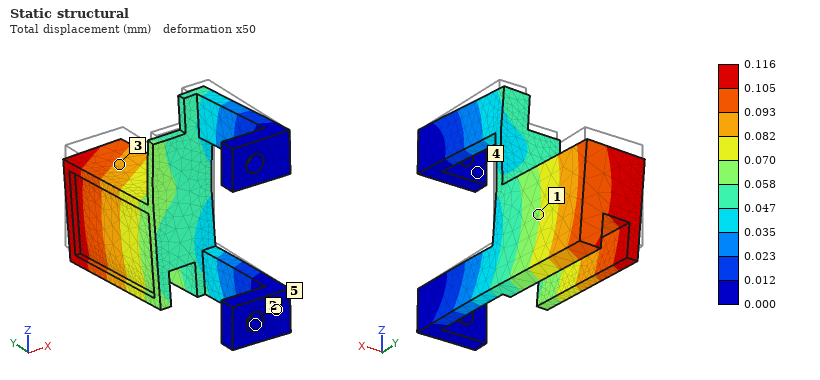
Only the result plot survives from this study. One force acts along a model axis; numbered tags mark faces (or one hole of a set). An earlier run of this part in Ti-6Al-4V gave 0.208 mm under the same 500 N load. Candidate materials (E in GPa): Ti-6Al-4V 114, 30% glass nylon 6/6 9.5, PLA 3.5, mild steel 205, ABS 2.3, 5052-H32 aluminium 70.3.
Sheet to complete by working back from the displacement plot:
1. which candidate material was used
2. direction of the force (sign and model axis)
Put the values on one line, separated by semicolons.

mild steel; -Z
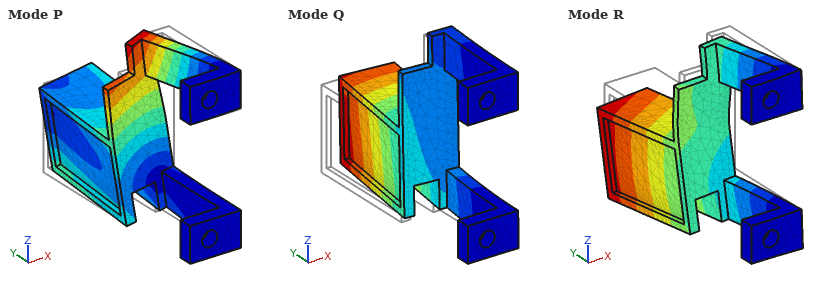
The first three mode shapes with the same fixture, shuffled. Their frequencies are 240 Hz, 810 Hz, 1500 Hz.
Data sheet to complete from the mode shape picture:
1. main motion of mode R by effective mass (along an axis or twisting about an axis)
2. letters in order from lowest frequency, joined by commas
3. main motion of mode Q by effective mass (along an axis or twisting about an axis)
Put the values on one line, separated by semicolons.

along Z; Q, R, P; along X
